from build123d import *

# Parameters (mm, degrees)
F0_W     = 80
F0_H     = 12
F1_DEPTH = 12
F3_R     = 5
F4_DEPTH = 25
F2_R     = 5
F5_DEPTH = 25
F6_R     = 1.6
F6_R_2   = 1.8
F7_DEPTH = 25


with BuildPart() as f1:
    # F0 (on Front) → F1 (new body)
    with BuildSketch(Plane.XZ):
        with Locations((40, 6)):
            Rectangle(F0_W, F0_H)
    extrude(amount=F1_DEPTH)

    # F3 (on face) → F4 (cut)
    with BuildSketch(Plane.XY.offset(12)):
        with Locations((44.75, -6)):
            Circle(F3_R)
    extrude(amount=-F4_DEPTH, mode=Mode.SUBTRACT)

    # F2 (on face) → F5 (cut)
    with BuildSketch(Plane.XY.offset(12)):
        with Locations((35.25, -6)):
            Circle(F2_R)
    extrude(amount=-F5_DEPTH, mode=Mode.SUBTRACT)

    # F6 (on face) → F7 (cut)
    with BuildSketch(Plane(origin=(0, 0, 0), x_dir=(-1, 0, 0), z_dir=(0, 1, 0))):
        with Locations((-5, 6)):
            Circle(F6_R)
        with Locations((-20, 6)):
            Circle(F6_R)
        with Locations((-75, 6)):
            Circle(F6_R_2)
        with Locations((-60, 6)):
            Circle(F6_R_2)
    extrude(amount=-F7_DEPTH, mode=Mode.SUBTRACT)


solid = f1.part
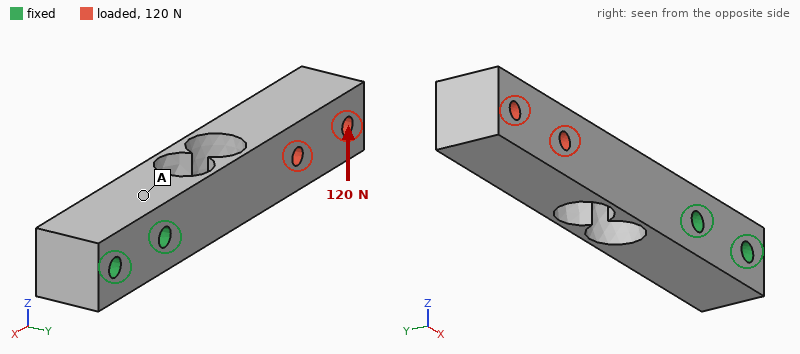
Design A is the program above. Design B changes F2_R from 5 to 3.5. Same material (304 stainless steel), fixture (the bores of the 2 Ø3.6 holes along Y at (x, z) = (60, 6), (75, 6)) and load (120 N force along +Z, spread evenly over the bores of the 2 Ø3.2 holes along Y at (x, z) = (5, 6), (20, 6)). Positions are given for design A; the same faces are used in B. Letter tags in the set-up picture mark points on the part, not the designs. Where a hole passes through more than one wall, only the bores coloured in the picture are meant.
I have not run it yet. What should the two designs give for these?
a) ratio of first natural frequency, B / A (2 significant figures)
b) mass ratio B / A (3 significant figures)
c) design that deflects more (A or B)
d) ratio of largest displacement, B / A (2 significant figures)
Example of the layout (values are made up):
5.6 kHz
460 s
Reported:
1.5
1.05
A
0.87
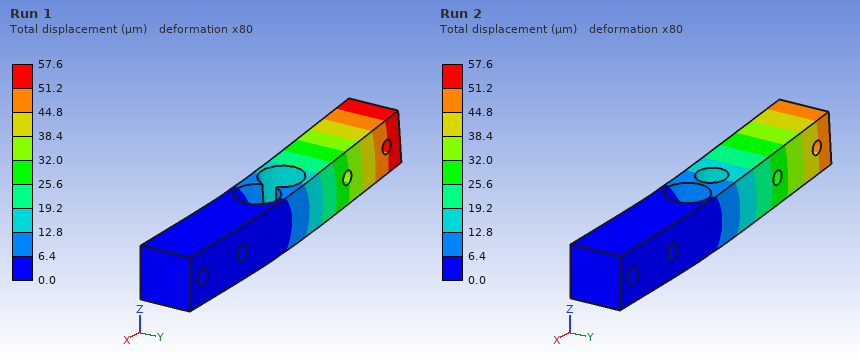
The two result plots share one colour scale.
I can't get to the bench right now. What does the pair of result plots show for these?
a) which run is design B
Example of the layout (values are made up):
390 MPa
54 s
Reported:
Run 2
